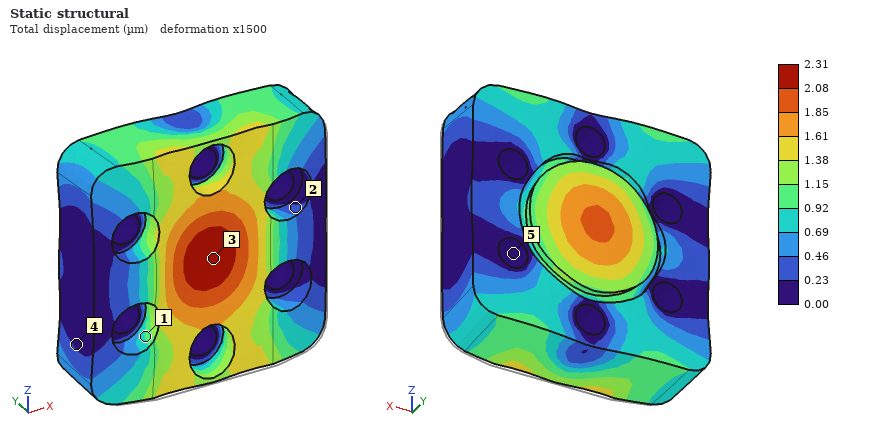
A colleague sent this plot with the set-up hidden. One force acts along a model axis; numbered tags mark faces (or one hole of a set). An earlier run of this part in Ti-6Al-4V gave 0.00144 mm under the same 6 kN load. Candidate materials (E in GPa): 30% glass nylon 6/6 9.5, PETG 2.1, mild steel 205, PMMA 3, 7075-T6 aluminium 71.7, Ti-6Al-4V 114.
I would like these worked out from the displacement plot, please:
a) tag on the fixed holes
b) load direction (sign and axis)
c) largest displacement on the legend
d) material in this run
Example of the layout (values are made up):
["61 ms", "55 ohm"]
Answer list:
["5", "+Y", "2.31 µm", "7075-T6 aluminium"]
